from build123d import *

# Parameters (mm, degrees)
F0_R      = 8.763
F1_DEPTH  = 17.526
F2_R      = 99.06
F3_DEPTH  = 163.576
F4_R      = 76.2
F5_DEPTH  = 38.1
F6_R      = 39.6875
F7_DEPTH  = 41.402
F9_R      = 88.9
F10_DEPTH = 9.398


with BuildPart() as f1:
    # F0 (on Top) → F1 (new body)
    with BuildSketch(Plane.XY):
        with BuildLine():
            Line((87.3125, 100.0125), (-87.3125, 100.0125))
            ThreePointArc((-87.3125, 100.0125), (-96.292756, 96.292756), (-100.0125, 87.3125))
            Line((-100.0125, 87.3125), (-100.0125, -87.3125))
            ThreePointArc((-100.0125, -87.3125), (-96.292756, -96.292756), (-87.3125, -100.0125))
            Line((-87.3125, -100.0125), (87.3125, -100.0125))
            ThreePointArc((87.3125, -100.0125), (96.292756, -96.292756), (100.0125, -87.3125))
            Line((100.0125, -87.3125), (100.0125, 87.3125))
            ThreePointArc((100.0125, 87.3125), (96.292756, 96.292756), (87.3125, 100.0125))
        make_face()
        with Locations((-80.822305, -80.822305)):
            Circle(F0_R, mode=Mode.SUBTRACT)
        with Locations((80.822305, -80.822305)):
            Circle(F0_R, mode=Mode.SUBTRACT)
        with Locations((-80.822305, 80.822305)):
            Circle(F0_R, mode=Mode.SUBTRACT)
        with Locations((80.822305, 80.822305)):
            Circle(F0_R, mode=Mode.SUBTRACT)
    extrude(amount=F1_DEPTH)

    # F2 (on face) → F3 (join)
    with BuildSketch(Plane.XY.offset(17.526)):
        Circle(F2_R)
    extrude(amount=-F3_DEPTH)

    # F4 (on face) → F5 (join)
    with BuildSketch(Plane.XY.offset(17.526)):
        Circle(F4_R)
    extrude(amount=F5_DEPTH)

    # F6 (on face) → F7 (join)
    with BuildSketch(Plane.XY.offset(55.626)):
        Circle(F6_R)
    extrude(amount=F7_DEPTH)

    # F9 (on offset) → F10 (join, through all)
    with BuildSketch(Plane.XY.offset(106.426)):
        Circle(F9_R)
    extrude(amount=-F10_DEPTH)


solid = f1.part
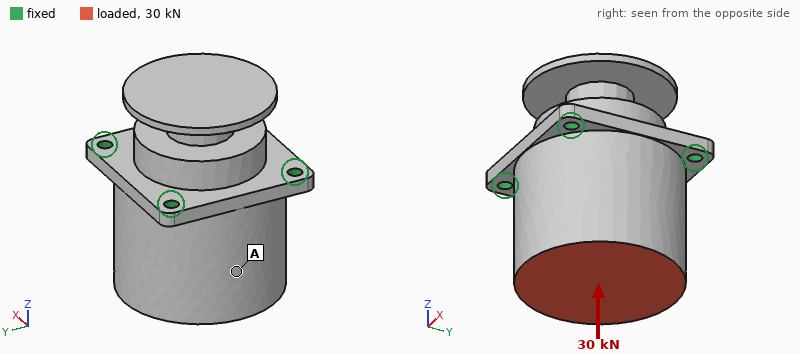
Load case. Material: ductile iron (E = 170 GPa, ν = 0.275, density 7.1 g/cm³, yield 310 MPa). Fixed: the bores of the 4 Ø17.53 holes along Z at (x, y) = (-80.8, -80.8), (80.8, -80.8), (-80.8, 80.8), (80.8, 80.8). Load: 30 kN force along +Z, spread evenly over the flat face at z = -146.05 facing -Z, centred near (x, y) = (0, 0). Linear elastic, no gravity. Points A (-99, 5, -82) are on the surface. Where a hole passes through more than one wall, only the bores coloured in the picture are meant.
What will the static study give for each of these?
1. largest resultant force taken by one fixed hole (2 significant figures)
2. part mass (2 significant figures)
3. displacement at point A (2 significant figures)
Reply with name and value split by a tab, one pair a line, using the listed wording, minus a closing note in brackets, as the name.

largest resultant force taken by one fixed hole	8.0 kN
part mass	45 kg
displacement at point A	5.3 µm
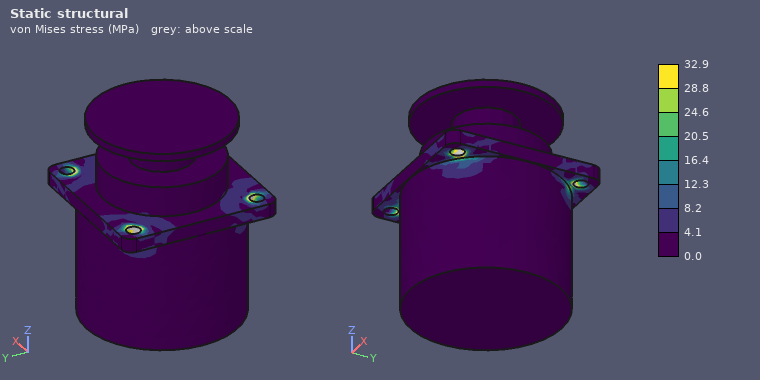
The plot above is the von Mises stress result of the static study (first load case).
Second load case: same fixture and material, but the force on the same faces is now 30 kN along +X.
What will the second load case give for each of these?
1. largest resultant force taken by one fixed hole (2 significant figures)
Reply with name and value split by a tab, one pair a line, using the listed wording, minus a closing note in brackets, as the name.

largest resultant force taken by one fixed hole	18 kN
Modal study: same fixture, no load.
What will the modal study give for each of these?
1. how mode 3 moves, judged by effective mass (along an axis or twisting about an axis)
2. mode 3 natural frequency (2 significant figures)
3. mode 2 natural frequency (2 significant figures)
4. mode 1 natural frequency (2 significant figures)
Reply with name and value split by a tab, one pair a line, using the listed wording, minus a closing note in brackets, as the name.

how mode 3 moves, judged by effective mass	along Z
mode 3 natural frequency	1800 Hz
mode 2 natural frequency	1400 Hz
mode 1 natural frequency	1400 Hz
